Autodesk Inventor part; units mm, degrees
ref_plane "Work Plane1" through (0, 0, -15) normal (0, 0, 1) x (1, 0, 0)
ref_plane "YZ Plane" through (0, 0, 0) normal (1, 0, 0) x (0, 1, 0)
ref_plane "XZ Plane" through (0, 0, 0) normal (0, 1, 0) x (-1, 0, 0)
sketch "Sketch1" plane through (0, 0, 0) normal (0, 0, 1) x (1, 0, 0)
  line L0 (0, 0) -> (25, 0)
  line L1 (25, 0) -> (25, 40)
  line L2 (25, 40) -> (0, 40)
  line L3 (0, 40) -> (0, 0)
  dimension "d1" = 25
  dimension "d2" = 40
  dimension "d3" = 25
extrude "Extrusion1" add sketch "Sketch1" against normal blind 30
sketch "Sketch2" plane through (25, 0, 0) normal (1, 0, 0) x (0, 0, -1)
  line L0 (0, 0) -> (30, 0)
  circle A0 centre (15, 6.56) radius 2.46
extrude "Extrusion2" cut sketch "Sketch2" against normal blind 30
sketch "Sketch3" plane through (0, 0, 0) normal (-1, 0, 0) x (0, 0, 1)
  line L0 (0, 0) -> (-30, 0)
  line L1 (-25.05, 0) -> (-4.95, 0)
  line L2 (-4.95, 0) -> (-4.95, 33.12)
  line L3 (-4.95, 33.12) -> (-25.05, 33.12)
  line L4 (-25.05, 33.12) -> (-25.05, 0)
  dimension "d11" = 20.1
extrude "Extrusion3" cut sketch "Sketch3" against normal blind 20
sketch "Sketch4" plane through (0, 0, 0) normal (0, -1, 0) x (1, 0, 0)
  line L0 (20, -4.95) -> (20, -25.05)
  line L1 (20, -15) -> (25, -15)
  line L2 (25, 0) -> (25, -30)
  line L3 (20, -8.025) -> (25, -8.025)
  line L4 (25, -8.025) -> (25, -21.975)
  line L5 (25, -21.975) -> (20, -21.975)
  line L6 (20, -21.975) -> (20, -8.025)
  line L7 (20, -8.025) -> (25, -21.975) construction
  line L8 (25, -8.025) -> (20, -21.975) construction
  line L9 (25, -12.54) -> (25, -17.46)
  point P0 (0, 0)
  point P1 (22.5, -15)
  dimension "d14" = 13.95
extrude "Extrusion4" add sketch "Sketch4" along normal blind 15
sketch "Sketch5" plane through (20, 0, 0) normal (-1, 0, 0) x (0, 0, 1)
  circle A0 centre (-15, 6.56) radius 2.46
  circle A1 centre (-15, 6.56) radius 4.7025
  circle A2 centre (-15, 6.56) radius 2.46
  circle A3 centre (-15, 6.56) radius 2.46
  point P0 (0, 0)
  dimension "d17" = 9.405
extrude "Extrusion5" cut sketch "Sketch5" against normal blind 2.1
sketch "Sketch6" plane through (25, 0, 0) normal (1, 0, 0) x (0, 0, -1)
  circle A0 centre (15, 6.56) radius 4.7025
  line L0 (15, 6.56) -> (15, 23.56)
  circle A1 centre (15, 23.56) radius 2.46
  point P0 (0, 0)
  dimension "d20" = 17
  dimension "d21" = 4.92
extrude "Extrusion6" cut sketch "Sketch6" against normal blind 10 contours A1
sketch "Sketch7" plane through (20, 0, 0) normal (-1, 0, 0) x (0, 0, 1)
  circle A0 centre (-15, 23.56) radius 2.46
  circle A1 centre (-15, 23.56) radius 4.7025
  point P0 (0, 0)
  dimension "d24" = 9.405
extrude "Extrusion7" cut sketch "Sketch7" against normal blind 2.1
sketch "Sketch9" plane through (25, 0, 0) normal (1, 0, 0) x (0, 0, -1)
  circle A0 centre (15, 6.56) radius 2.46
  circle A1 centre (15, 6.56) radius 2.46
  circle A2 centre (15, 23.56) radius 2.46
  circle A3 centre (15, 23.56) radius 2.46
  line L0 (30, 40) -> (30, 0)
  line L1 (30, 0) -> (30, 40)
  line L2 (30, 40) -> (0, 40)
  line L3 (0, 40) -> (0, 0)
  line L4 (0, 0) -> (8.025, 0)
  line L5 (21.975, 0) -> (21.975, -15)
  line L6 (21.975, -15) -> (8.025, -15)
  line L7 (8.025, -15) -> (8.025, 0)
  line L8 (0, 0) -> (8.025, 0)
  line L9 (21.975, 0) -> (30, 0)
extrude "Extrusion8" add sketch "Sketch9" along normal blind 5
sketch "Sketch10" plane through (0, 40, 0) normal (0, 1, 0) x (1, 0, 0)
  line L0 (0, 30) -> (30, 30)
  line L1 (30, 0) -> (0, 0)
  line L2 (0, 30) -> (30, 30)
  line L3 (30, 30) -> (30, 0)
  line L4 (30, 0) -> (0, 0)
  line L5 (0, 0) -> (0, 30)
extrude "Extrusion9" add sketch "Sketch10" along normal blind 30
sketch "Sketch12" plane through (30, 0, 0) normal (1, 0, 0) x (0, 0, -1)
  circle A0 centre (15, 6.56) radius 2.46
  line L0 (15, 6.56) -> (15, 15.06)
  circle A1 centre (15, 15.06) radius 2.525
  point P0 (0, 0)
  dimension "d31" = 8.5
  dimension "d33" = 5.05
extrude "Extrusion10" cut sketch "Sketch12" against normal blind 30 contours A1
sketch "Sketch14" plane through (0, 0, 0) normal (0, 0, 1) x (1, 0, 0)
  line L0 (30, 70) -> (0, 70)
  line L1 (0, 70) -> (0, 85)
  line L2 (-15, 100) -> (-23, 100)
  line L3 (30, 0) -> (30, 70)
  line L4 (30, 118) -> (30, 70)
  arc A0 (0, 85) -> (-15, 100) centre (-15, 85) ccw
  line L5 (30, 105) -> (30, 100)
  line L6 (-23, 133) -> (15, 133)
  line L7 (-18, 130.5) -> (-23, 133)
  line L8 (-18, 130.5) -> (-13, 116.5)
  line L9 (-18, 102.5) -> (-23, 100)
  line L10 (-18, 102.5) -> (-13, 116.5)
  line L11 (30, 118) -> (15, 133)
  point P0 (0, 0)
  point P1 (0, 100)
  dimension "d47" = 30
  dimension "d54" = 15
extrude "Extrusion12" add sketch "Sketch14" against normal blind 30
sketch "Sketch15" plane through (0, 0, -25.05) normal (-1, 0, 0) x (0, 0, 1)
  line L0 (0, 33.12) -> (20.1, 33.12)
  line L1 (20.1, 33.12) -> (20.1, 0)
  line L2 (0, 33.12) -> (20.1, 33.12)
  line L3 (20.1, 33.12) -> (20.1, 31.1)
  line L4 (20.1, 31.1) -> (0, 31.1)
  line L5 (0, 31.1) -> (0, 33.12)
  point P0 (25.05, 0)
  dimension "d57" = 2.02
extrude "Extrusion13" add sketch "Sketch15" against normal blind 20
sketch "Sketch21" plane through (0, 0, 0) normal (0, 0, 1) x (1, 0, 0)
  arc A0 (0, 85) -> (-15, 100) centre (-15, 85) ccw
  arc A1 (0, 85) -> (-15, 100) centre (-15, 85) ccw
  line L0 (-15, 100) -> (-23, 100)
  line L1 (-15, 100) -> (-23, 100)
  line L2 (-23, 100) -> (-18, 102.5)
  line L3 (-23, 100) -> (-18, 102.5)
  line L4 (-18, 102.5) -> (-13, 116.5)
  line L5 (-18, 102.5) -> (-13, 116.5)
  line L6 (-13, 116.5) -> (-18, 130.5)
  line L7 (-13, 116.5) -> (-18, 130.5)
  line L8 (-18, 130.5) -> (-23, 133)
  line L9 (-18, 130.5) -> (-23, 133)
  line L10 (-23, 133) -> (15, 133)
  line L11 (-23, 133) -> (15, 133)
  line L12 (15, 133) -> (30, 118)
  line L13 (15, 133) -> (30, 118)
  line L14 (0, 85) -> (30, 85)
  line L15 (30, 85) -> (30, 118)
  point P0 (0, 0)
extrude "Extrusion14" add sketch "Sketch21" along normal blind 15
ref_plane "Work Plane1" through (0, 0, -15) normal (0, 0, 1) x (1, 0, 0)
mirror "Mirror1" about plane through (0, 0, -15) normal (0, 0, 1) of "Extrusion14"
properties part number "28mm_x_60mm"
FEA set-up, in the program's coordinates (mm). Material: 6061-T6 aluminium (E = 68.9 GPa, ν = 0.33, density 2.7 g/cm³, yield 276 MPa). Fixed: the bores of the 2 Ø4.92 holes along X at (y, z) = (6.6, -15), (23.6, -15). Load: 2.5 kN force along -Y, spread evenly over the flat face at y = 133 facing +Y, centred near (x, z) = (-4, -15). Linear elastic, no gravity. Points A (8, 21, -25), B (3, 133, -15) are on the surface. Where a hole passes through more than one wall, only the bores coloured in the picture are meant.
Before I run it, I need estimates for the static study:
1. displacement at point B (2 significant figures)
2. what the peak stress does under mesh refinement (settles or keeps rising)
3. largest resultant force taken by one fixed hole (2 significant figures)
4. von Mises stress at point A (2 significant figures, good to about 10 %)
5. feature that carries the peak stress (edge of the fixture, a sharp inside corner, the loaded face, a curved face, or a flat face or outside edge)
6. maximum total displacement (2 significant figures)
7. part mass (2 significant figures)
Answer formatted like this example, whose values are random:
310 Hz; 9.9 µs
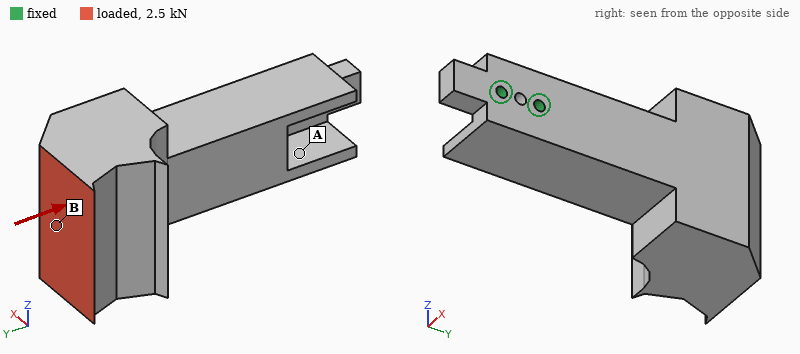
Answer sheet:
0.23 mm; keeps rising; 3.4 kN; 23 MPa; edge of the fixture; 0.25 mm; 490 g
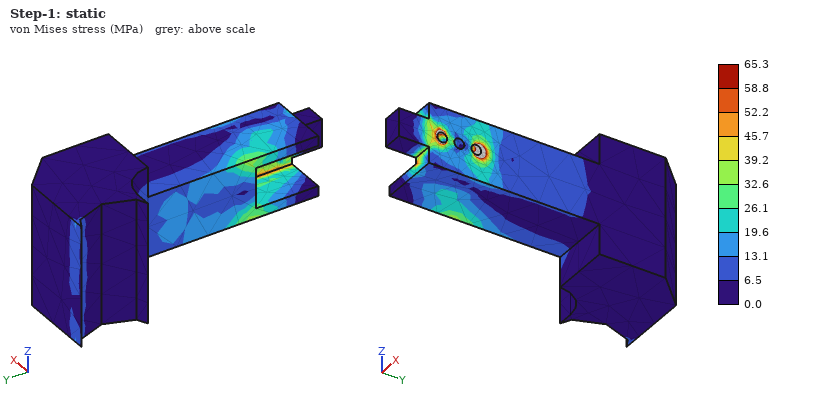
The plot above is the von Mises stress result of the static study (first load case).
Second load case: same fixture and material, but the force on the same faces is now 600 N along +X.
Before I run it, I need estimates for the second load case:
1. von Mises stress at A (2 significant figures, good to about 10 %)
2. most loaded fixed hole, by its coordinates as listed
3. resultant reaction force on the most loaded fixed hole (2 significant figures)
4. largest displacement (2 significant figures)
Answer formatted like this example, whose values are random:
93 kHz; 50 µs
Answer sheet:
19 MPa; (23.6, -15); 3.2 kN; 0.23 mm
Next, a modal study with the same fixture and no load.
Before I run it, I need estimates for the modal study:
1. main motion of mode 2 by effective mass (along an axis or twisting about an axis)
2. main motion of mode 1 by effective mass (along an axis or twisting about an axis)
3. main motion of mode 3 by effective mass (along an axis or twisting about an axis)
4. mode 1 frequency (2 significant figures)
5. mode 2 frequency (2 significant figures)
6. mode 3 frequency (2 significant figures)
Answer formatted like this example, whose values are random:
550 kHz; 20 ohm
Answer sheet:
along Z; along X; twisting about Y; 590 Hz; 680 Hz; 1600 Hz
